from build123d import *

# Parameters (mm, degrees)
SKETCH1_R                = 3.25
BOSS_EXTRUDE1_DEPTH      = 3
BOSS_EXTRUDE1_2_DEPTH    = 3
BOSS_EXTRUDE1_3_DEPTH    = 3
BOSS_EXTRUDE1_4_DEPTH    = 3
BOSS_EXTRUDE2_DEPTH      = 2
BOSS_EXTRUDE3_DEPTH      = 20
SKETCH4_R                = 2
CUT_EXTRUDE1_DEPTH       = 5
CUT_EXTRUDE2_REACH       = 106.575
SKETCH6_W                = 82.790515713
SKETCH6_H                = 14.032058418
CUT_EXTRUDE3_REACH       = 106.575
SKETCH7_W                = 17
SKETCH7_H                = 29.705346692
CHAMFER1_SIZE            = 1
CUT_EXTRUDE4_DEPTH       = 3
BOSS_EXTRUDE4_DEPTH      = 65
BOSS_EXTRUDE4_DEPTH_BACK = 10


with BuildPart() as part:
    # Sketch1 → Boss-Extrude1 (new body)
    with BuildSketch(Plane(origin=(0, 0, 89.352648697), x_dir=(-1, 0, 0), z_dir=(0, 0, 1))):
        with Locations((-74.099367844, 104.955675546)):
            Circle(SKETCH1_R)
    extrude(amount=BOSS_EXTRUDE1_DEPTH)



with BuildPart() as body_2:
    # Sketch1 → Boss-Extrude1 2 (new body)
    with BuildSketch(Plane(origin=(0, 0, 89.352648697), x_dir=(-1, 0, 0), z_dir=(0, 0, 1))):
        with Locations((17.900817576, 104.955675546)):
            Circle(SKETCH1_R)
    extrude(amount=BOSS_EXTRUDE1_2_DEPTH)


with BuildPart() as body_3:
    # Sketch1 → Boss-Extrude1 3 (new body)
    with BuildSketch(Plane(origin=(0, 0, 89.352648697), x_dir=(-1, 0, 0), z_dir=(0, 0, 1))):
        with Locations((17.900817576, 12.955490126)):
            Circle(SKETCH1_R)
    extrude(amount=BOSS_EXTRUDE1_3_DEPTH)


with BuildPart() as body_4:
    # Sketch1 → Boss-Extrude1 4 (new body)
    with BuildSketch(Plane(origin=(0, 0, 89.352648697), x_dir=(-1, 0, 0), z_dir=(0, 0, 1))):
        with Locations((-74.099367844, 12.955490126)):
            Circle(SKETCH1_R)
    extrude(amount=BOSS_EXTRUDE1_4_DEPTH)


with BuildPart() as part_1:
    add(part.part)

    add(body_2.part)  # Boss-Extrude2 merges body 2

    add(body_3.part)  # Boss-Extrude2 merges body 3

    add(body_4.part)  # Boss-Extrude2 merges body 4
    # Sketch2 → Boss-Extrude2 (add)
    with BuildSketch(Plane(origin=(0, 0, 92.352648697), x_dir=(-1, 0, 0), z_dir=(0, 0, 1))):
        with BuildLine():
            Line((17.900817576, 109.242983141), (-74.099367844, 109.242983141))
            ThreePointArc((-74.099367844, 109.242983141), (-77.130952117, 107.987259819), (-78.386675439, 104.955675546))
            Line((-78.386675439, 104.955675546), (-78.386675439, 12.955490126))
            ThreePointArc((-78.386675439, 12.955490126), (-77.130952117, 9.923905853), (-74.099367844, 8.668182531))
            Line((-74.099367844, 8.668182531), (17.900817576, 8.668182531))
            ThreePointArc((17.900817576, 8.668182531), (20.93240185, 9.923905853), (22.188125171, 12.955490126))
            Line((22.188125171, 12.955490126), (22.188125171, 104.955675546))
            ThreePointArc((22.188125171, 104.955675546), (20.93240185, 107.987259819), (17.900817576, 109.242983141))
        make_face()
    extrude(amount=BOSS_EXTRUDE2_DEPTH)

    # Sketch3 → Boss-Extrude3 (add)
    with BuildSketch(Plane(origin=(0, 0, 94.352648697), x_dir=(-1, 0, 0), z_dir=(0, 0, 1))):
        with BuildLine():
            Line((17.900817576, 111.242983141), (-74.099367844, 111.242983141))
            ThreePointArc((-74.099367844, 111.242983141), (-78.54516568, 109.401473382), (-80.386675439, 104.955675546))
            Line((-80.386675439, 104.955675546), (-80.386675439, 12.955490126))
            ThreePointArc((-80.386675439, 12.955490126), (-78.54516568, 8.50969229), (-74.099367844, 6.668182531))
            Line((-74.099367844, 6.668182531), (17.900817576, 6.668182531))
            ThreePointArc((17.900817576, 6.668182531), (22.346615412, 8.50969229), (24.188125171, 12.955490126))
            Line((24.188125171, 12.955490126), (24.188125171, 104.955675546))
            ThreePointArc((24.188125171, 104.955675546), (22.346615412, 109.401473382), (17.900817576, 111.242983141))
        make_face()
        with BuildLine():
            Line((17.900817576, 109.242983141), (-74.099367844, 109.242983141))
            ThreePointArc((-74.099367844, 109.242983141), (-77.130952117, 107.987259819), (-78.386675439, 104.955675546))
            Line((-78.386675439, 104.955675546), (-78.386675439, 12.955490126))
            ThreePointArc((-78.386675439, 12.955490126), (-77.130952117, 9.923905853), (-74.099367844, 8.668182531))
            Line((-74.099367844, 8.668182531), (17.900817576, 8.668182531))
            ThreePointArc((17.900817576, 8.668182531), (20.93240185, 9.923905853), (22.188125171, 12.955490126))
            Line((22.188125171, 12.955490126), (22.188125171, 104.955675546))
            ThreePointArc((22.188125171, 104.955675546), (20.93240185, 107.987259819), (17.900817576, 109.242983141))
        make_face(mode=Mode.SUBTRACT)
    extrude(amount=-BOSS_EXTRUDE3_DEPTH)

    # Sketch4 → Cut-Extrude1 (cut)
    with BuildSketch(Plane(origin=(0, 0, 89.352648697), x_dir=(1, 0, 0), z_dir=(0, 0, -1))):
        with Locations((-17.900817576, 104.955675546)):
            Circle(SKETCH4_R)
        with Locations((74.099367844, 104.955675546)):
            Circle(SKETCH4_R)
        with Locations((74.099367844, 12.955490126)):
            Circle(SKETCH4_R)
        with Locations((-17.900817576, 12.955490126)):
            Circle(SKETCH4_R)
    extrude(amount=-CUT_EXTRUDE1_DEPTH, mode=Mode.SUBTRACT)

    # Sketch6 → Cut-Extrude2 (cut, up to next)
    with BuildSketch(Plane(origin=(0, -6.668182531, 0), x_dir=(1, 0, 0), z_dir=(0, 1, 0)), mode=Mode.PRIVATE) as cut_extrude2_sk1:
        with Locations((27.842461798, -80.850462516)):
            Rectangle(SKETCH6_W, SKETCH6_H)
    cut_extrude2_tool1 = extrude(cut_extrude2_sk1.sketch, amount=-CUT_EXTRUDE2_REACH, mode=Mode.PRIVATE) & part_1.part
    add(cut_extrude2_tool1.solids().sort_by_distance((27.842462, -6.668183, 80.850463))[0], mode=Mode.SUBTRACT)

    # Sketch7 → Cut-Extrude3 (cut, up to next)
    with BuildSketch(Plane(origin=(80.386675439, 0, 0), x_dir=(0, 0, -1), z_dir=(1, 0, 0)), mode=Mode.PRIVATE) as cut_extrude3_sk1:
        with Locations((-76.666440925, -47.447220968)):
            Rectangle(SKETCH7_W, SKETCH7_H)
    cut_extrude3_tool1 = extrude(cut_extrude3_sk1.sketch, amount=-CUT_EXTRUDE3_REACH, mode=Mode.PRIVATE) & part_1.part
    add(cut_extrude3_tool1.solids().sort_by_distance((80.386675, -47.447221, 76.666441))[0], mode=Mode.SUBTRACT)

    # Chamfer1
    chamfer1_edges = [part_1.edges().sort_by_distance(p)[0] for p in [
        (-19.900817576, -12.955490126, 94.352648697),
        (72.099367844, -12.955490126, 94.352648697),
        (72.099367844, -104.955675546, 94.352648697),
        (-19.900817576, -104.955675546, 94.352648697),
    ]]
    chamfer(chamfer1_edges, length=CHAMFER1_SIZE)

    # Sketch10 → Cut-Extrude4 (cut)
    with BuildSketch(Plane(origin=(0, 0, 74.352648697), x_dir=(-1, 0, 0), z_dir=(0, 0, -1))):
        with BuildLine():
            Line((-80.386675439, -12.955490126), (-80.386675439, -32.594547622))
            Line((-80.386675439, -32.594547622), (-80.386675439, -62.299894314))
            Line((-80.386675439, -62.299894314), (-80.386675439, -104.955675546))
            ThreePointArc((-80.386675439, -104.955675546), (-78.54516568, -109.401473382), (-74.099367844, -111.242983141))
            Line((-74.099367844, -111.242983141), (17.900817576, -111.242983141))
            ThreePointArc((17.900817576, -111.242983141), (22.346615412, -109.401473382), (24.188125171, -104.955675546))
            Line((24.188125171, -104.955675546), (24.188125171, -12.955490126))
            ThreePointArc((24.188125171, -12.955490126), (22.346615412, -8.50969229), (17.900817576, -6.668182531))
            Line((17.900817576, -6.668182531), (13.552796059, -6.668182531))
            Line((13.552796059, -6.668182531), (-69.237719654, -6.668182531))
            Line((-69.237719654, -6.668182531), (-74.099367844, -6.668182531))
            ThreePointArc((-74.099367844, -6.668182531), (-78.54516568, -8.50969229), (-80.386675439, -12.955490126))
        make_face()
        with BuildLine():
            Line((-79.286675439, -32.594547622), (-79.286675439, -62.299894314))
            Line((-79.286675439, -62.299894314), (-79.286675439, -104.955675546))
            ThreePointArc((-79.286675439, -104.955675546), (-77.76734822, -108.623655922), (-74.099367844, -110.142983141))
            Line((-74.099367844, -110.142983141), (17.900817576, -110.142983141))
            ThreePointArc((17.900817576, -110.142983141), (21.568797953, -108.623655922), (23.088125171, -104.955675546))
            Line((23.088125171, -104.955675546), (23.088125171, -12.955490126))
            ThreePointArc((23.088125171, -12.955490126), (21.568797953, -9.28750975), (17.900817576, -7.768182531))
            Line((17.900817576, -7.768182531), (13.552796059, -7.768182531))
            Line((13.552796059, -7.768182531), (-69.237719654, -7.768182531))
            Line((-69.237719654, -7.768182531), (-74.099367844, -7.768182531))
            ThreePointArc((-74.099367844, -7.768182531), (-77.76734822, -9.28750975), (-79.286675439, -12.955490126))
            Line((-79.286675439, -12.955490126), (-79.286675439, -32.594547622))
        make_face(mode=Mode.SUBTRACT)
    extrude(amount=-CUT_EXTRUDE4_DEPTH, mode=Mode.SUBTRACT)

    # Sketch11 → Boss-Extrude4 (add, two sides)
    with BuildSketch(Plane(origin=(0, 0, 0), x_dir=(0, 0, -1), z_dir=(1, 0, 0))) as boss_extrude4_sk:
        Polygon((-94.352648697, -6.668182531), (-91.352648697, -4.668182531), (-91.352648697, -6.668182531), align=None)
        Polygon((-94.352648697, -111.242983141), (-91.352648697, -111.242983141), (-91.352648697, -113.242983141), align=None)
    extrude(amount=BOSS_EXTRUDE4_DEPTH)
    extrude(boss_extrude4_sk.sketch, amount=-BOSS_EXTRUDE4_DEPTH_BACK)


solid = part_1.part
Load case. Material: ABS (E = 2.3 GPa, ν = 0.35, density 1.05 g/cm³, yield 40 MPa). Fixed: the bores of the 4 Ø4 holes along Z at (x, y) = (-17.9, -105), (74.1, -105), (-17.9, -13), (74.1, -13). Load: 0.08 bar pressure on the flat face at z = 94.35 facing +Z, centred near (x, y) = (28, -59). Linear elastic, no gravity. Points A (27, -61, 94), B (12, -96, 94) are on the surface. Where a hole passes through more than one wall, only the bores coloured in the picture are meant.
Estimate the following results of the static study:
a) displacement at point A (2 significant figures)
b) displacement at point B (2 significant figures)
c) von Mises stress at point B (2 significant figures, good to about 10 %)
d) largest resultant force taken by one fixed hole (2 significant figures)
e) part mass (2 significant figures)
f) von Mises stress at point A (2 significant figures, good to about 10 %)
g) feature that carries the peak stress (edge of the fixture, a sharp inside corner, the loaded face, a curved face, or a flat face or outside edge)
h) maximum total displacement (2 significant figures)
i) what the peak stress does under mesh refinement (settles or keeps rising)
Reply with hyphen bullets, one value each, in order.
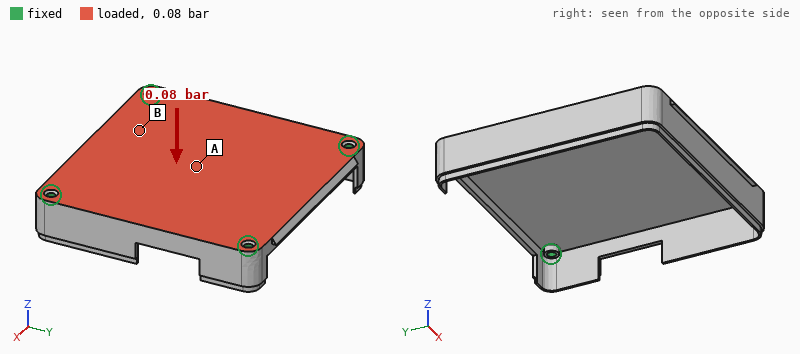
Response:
- 1.4 mm
- 0.50 mm
- 2.2 MPa
- 23 N
- 35 g
- 4.8 MPa
- edge of the fixture
- 1.5 mm
- keeps rising
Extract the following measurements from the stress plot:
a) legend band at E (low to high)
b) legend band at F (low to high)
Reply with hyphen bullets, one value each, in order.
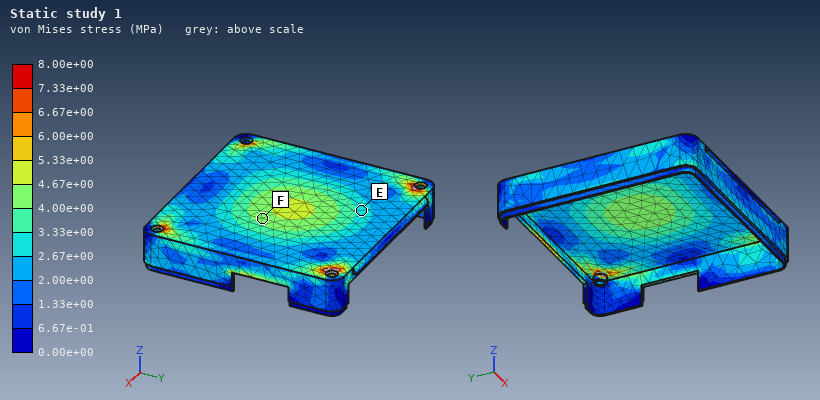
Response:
- 2.67e+00 to 3.33e+00 MPa
- 4.00e+00 to 4.67e+00 MPa
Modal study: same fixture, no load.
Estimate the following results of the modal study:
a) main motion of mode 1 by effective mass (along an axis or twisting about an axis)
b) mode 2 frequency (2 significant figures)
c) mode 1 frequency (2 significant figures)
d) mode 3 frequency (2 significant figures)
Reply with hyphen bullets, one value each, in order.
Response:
- along Z
- 630 Hz
- 320 Hz
- 680 Hz
